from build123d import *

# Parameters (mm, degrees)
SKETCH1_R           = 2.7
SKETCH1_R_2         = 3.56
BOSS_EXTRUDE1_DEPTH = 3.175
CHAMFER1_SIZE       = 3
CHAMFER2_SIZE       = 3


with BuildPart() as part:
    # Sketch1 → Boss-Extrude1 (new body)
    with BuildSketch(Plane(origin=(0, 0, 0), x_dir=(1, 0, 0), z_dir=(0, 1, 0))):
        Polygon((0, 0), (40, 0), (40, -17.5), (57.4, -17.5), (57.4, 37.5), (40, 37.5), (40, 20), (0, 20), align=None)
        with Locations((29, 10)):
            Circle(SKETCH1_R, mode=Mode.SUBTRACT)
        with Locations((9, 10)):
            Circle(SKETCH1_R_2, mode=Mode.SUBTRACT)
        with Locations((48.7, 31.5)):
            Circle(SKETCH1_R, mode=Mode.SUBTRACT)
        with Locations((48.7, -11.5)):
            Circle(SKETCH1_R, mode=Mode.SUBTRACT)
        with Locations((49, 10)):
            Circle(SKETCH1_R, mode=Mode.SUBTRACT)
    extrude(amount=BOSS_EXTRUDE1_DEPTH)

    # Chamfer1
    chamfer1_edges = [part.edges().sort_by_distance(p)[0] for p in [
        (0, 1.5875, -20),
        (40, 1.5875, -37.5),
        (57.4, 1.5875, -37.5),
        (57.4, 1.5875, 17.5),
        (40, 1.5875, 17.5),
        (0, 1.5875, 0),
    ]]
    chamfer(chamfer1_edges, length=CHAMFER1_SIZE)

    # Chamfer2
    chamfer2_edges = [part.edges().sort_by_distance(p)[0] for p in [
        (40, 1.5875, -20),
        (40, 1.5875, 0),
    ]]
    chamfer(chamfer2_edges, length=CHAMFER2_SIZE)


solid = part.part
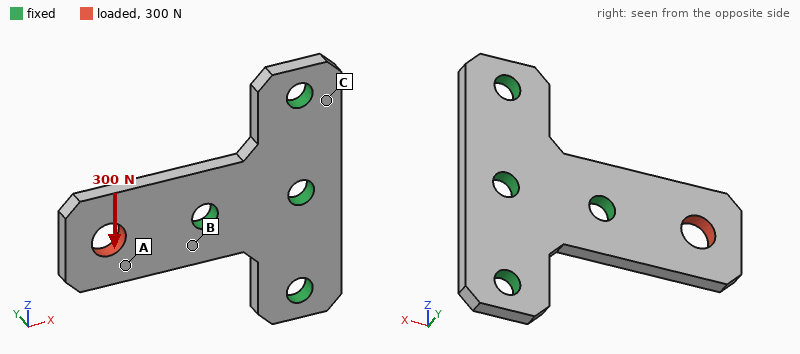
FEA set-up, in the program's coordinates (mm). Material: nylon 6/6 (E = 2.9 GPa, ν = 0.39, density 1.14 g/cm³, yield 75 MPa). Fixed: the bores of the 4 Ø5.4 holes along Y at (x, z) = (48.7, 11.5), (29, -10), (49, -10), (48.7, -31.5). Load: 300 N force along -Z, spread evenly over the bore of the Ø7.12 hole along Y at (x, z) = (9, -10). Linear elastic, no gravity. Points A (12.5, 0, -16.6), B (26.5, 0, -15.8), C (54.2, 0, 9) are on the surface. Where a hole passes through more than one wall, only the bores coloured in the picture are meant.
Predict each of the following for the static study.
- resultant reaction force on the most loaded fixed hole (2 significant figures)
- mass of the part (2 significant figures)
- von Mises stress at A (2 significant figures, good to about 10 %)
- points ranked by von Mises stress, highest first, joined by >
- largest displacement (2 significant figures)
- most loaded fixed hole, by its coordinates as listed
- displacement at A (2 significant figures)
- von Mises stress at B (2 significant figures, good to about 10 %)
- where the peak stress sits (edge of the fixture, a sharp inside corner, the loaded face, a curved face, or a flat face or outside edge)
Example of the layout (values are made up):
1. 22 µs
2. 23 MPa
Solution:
1. 440 N
2. 5.8 g
3. 8.9 MPa
4. B > A > C
5. 0.56 mm
6. (29, -10)
7. 0.30 mm
8. 15 MPa
9. edge of the fixture
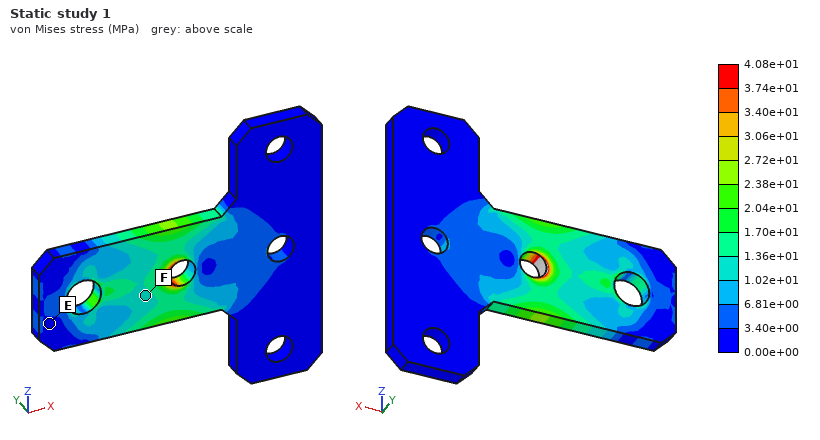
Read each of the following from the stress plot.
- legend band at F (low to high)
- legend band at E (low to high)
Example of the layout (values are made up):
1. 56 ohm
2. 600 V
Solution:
1. 1.02e+01 to 1.36e+01 MPa
2. 0.00e+00 to 3.40e+00 MPa
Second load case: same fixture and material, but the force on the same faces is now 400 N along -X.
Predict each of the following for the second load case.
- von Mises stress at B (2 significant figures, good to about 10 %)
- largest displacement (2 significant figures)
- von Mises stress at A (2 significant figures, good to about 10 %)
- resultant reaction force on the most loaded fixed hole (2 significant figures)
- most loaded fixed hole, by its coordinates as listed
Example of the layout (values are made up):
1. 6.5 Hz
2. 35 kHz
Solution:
1. 4.3 MPa
2. 80 µm
3. 7.1 MPa
4. 330 N
5. (29, -10)
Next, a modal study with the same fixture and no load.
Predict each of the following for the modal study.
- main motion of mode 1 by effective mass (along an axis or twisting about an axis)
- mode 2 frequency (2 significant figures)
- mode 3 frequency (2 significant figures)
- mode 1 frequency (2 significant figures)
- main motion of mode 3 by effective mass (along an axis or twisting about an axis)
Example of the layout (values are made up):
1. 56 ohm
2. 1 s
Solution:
1. along Y
2. 2800 Hz
3. 3900 Hz
4. 1200 Hz
5. along Z
